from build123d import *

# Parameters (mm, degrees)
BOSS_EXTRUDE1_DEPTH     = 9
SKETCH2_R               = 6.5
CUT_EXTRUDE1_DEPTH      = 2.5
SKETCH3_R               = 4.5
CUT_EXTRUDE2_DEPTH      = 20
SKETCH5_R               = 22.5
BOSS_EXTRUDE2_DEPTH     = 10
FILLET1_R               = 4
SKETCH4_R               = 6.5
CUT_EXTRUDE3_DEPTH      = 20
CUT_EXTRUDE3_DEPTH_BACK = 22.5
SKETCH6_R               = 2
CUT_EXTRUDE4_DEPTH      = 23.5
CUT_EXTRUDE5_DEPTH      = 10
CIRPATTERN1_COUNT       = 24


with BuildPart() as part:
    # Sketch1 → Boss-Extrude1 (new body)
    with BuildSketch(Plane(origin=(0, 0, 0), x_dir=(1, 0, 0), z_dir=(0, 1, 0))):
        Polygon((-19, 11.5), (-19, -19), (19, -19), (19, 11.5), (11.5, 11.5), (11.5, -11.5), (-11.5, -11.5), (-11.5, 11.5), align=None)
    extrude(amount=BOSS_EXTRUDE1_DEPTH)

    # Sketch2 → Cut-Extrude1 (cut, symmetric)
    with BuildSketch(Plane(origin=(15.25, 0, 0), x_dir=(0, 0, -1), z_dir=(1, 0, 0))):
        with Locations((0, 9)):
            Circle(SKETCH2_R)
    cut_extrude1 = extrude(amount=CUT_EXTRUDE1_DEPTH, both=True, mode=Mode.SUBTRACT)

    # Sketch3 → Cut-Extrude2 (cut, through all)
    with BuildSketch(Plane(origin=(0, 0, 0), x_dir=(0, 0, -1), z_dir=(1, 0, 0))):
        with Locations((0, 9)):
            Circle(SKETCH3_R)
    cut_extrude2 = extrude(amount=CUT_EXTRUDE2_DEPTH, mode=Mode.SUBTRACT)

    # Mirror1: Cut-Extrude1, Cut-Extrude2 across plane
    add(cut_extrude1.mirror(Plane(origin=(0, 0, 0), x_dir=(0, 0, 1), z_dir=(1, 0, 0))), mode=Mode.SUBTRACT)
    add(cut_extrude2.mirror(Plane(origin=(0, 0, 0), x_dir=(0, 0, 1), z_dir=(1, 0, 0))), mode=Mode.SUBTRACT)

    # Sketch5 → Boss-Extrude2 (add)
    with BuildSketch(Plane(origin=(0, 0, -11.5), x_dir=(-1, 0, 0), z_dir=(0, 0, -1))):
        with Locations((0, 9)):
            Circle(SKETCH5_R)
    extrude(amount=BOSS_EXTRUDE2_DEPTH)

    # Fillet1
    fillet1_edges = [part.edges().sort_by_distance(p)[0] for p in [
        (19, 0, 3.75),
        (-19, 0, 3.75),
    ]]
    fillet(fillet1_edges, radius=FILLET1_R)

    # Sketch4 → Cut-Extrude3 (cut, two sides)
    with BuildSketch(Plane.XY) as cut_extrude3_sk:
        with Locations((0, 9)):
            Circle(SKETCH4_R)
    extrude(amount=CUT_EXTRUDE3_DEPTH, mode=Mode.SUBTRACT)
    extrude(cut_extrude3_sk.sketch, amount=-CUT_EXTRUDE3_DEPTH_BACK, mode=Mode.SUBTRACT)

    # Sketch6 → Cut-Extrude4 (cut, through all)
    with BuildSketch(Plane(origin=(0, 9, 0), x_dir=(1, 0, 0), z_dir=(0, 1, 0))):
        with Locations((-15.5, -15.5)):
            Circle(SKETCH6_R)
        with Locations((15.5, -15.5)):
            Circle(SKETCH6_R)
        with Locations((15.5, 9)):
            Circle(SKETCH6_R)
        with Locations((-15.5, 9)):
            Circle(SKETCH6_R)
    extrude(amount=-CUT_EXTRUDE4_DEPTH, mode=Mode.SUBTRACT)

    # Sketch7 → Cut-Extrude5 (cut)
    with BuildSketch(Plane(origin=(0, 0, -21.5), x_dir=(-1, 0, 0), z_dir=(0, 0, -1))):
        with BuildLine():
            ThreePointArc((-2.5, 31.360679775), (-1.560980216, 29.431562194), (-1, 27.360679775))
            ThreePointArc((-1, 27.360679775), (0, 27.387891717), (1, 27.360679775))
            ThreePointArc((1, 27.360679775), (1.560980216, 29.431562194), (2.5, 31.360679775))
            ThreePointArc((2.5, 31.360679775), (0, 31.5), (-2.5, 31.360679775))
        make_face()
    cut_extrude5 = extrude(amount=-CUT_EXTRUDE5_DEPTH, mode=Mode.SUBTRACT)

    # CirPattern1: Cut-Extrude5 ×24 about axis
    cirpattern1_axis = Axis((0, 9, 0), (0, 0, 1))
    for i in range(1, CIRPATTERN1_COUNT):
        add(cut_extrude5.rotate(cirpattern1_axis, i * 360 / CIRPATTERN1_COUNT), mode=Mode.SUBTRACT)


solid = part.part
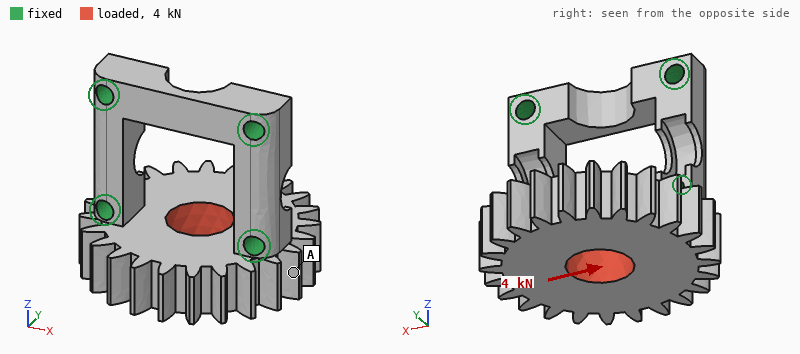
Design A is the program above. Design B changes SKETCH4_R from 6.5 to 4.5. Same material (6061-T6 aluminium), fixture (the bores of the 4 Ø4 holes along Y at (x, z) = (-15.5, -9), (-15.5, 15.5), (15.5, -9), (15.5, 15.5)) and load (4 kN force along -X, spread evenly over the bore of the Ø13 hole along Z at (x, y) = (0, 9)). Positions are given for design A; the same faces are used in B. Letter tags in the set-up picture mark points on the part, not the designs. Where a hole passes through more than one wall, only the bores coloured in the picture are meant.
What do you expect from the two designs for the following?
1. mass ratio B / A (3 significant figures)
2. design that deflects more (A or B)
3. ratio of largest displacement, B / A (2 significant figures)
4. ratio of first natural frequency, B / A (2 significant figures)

1.06
A
0.85
1.00
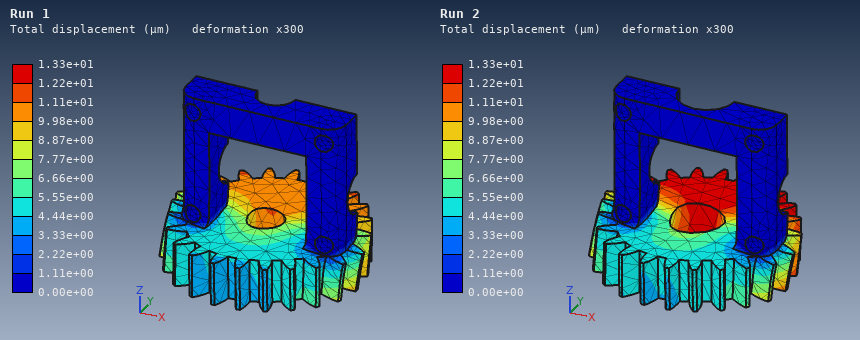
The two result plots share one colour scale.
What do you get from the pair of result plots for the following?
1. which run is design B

Run 1
